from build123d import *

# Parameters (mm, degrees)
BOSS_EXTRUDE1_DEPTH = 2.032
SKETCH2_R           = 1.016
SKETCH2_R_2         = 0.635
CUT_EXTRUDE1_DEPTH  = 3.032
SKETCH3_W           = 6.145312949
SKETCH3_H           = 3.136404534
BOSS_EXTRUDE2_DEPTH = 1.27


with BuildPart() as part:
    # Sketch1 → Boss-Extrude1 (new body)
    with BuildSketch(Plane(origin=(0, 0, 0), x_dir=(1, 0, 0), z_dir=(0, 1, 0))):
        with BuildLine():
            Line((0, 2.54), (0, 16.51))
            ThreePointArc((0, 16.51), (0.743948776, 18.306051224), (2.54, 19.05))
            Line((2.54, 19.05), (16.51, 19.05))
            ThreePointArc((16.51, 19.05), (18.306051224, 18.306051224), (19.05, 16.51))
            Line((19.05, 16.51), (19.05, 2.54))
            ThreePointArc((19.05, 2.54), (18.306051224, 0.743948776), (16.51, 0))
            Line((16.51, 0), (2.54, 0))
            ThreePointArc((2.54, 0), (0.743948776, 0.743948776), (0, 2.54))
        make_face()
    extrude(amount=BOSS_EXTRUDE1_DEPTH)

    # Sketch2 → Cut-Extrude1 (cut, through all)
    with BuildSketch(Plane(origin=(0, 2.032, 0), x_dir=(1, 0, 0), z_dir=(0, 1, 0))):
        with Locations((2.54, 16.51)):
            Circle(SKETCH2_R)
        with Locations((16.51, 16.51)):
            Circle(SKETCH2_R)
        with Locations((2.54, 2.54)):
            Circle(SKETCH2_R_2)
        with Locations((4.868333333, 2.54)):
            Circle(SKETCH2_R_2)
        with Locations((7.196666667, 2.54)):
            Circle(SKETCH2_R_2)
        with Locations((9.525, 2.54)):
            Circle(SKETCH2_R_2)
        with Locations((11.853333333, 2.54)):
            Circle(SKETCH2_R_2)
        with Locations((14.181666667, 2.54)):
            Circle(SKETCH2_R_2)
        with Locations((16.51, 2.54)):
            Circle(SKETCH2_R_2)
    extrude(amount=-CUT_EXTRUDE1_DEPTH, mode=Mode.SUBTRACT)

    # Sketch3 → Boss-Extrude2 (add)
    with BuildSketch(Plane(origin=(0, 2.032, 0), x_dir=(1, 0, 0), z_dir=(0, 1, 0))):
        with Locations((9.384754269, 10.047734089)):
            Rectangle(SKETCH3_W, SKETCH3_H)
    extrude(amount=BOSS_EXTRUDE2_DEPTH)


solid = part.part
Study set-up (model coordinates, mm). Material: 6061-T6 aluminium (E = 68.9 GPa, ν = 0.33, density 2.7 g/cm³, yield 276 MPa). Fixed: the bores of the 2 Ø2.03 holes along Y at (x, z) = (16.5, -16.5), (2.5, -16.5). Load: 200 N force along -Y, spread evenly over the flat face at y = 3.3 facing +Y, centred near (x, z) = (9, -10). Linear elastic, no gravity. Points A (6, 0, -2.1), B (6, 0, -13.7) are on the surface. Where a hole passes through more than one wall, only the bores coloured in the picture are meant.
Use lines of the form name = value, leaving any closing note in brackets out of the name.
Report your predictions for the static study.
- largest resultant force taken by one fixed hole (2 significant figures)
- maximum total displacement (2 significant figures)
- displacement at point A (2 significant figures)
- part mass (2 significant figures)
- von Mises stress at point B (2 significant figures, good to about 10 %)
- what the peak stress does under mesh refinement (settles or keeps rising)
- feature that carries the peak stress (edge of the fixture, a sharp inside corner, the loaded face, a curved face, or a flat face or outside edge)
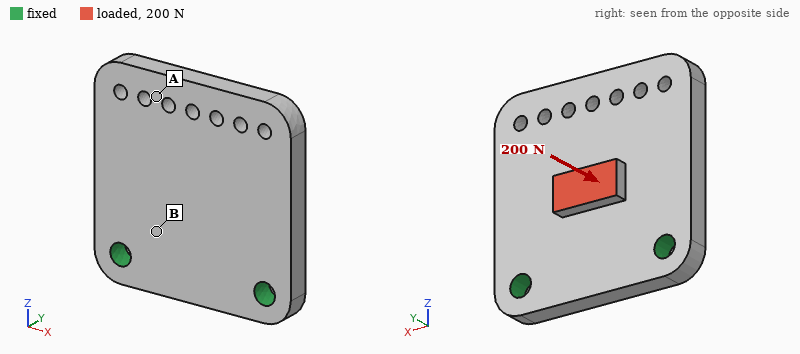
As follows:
largest resultant force taken by one fixed hole = 100 N
maximum total displacement = 86 µm
displacement at point A = 73 µm
part mass = 1.9 g
von Mises stress at point B = 46 MPa
what the peak stress does under mesh refinement = keeps rising
feature that carries the peak stress = edge of the fixture
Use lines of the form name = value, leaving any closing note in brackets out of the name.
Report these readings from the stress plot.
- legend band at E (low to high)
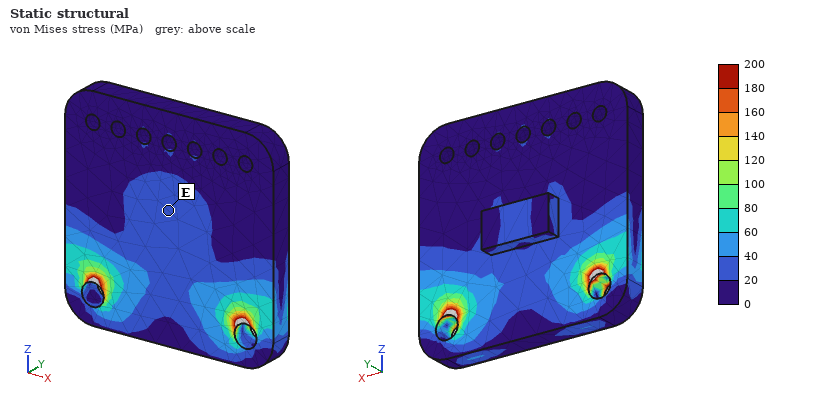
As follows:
legend band at E = 20 to 40 MPa
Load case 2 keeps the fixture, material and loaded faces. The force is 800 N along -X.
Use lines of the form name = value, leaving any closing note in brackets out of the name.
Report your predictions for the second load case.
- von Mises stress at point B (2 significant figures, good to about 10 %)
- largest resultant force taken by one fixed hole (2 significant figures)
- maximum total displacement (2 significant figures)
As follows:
von Mises stress at point B = 30 MPa
largest resultant force taken by one fixed hole = 540 N
maximum total displacement = 35 µm
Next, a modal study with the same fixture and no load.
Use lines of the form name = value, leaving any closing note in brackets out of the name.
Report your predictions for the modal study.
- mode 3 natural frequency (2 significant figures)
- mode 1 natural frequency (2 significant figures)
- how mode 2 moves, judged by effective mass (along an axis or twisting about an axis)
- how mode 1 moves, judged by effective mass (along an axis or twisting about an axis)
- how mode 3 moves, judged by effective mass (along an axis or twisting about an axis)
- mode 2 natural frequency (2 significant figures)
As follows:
mode 3 natural frequency = 34 kHz
mode 1 natural frequency = 6100 Hz
how mode 2 moves, judged by effective mass = twisting about Z
how mode 1 moves, judged by effective mass = along Y
how mode 3 moves, judged by effective mass = along Y
mode 2 natural frequency = 14 kHz
